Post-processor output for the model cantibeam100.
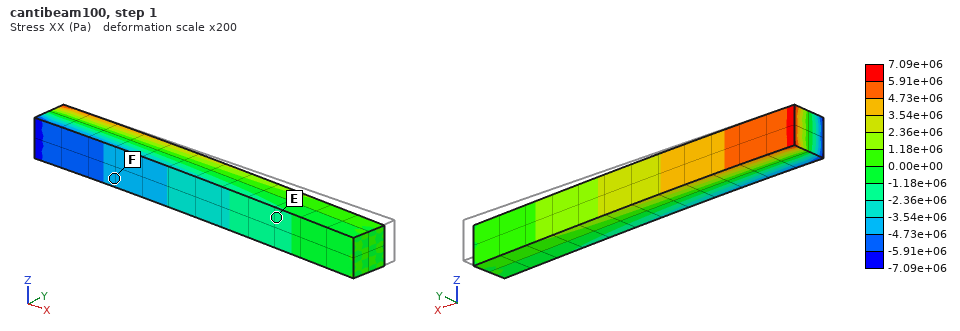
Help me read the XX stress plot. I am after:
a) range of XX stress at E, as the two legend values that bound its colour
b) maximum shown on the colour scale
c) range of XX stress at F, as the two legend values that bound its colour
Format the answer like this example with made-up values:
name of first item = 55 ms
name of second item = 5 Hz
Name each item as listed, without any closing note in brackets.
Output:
range of XX stress at E, as the two legend values that bound its colour = -2.36e+06 to -1.18e+06 Pa
maximum shown on the colour scale = 7.09e+06 Pa
range of XX stress at F, as the two legend values that bound its colour = -4.73e+06 to -3.54e+06 Pa
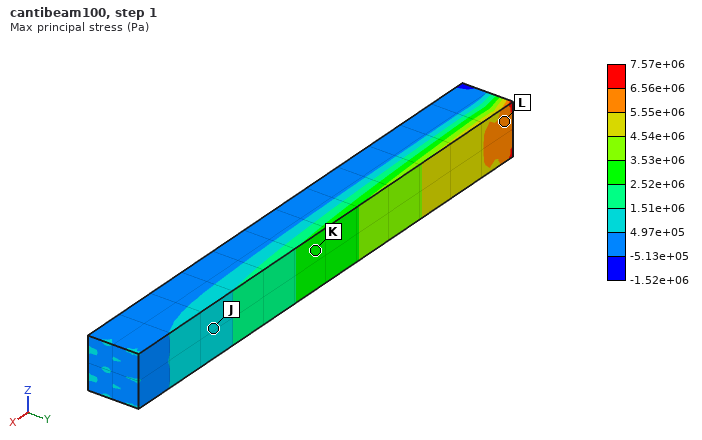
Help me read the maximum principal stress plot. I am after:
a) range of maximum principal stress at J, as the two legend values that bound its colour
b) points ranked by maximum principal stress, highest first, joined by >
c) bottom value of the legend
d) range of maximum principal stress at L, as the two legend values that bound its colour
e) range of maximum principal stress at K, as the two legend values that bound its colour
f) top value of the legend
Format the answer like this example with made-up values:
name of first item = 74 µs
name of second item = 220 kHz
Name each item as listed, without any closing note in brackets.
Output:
range of maximum principal stress at J, as the two legend values that bound its colour = 4.97e+05 to 1.51e+06 Pa
points ranked by maximum principal stress, highest first, joined by > = L > K > J
bottom value of the legend = -1.52e+06 Pa
range of maximum principal stress at L, as the two legend values that bound its colour = 5.55e+06 to 6.56e+06 Pa
range of maximum principal stress at K, as the two legend values that bound its colour = 2.52e+06 to 3.53e+06 Pa
top value of the legend = 7.57e+06 Pa
